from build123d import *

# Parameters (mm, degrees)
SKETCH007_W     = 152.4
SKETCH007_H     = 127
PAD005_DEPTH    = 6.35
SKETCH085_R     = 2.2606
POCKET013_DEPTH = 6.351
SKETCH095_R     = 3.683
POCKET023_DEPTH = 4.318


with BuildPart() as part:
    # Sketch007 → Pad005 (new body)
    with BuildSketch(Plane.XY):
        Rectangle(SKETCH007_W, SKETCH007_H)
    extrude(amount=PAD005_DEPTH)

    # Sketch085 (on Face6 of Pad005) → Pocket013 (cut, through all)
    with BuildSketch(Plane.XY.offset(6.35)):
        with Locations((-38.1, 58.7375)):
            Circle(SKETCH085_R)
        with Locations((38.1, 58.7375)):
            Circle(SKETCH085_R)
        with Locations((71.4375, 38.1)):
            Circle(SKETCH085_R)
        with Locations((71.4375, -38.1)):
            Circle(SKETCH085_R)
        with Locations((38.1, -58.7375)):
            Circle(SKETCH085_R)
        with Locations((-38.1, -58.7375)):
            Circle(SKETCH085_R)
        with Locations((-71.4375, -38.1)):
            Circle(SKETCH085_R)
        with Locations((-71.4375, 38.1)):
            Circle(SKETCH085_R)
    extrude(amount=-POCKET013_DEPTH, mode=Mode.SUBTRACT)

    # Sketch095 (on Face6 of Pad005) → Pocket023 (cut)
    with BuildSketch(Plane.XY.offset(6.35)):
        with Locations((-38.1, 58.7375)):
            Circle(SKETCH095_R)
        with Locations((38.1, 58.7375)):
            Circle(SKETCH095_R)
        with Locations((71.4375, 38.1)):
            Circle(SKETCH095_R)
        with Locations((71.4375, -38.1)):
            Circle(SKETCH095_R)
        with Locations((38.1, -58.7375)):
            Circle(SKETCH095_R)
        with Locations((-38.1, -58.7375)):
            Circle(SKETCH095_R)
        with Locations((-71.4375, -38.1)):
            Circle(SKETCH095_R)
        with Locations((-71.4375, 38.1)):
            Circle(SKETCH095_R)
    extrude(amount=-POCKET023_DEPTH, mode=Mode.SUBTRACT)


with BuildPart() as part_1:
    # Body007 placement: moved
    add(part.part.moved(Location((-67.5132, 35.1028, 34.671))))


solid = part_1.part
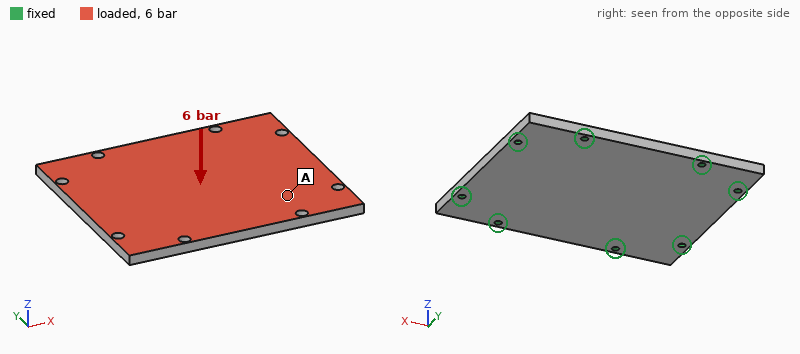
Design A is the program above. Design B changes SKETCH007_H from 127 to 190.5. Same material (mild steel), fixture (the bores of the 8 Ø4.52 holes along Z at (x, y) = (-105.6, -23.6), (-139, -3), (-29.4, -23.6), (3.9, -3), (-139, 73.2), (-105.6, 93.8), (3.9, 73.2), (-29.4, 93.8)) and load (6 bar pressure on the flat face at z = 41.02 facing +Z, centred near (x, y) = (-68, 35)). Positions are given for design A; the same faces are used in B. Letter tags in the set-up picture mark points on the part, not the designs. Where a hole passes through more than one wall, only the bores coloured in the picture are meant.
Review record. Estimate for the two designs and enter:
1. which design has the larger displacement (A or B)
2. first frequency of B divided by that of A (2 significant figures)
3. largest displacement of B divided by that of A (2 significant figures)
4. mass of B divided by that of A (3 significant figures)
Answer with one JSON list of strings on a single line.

["A", "0.90", "0.66", "1.51"]
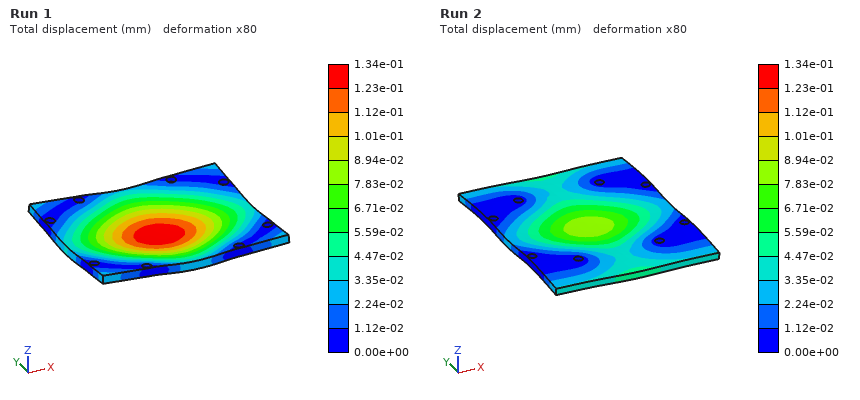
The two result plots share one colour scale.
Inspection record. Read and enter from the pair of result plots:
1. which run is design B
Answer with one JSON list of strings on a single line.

["Run 2"]
